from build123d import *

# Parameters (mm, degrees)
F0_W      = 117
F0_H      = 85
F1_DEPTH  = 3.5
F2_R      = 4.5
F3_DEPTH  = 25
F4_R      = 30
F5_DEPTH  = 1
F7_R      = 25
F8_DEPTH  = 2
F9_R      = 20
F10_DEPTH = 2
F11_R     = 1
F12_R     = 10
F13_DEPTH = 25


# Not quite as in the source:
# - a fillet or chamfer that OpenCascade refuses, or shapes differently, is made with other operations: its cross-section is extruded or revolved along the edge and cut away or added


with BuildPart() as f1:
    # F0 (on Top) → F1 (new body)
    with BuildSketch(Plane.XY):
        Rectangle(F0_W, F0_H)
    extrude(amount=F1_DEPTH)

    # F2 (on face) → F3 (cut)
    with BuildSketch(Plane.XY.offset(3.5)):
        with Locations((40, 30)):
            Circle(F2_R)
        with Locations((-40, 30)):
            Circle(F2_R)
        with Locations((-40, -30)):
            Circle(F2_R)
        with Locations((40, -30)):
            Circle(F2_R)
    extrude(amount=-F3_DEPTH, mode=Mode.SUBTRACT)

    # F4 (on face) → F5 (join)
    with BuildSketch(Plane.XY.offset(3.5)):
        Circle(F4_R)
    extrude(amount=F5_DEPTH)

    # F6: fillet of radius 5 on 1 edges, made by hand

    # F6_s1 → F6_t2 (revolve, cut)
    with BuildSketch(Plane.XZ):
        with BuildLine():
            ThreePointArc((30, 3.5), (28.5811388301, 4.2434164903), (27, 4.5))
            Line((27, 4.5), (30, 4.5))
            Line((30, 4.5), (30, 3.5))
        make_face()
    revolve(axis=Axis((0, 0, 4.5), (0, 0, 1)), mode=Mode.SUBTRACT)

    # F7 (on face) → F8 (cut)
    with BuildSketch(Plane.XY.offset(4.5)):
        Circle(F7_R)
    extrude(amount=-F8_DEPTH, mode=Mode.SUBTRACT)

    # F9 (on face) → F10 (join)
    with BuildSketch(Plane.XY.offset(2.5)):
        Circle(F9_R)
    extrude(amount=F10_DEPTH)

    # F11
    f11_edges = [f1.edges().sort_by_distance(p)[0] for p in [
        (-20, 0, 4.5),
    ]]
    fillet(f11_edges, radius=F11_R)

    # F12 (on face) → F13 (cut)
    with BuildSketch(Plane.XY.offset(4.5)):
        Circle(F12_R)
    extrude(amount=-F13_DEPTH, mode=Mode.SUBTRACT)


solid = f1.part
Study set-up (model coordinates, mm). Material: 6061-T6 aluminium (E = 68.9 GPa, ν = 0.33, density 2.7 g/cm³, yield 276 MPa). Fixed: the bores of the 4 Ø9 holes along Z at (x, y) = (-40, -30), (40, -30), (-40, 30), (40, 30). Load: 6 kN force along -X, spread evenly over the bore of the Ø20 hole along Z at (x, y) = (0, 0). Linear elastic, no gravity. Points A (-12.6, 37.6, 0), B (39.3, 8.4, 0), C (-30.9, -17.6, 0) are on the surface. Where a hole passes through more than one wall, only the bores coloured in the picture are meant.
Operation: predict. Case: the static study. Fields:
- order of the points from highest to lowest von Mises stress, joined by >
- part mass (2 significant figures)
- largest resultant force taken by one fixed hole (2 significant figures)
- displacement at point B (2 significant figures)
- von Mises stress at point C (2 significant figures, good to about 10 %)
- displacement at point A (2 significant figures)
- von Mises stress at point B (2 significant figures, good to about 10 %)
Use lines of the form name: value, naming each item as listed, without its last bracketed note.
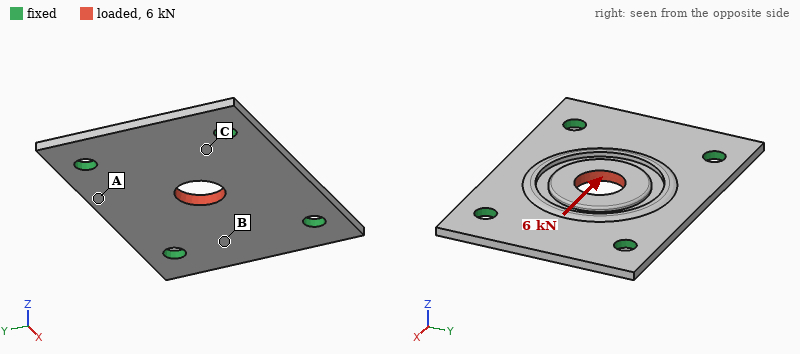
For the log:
order of the points from highest to lowest von Mises stress, joined by >: C > B > A
part mass: 91 g
largest resultant force taken by one fixed hole: 1.6 kN
displacement at point B: 7.6 µm
von Mises stress at point C: 21 MPa
displacement at point A: 3.1 µm
von Mises stress at point B: 11 MPa
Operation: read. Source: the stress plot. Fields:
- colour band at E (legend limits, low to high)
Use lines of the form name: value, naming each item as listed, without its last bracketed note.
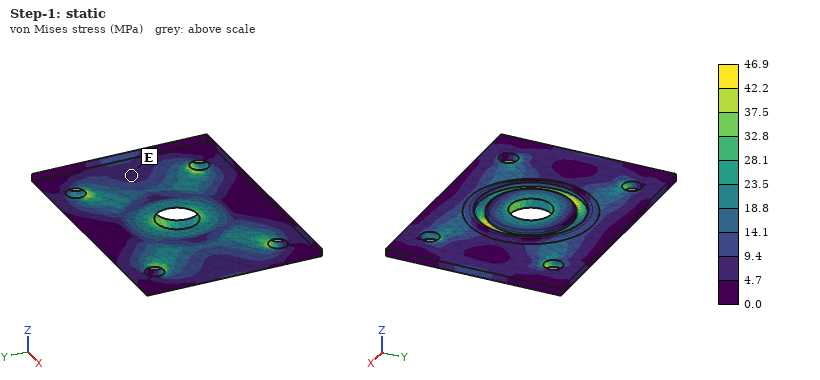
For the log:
colour band at E: 4.7 to 9.4 MPa
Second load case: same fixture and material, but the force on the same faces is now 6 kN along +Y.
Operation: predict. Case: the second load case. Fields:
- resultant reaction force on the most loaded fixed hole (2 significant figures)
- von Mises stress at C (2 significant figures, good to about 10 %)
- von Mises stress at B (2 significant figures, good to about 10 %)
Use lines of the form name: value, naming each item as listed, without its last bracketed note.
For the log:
resultant reaction force on the most loaded fixed hole: 1.7 kN
von Mises stress at C: 22 MPa
von Mises stress at B: 8.2 MPa
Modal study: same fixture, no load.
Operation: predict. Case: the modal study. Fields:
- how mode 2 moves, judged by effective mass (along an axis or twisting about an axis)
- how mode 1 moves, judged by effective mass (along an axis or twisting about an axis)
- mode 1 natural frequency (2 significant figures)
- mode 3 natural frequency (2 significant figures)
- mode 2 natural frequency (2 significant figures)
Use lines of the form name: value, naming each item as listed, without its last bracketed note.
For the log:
how mode 2 moves, judged by effective mass: twisting about X
how mode 1 moves, judged by effective mass: along Z
mode 1 natural frequency: 2900 Hz
mode 3 natural frequency: 4900 Hz
mode 2 natural frequency: 3700 Hz
